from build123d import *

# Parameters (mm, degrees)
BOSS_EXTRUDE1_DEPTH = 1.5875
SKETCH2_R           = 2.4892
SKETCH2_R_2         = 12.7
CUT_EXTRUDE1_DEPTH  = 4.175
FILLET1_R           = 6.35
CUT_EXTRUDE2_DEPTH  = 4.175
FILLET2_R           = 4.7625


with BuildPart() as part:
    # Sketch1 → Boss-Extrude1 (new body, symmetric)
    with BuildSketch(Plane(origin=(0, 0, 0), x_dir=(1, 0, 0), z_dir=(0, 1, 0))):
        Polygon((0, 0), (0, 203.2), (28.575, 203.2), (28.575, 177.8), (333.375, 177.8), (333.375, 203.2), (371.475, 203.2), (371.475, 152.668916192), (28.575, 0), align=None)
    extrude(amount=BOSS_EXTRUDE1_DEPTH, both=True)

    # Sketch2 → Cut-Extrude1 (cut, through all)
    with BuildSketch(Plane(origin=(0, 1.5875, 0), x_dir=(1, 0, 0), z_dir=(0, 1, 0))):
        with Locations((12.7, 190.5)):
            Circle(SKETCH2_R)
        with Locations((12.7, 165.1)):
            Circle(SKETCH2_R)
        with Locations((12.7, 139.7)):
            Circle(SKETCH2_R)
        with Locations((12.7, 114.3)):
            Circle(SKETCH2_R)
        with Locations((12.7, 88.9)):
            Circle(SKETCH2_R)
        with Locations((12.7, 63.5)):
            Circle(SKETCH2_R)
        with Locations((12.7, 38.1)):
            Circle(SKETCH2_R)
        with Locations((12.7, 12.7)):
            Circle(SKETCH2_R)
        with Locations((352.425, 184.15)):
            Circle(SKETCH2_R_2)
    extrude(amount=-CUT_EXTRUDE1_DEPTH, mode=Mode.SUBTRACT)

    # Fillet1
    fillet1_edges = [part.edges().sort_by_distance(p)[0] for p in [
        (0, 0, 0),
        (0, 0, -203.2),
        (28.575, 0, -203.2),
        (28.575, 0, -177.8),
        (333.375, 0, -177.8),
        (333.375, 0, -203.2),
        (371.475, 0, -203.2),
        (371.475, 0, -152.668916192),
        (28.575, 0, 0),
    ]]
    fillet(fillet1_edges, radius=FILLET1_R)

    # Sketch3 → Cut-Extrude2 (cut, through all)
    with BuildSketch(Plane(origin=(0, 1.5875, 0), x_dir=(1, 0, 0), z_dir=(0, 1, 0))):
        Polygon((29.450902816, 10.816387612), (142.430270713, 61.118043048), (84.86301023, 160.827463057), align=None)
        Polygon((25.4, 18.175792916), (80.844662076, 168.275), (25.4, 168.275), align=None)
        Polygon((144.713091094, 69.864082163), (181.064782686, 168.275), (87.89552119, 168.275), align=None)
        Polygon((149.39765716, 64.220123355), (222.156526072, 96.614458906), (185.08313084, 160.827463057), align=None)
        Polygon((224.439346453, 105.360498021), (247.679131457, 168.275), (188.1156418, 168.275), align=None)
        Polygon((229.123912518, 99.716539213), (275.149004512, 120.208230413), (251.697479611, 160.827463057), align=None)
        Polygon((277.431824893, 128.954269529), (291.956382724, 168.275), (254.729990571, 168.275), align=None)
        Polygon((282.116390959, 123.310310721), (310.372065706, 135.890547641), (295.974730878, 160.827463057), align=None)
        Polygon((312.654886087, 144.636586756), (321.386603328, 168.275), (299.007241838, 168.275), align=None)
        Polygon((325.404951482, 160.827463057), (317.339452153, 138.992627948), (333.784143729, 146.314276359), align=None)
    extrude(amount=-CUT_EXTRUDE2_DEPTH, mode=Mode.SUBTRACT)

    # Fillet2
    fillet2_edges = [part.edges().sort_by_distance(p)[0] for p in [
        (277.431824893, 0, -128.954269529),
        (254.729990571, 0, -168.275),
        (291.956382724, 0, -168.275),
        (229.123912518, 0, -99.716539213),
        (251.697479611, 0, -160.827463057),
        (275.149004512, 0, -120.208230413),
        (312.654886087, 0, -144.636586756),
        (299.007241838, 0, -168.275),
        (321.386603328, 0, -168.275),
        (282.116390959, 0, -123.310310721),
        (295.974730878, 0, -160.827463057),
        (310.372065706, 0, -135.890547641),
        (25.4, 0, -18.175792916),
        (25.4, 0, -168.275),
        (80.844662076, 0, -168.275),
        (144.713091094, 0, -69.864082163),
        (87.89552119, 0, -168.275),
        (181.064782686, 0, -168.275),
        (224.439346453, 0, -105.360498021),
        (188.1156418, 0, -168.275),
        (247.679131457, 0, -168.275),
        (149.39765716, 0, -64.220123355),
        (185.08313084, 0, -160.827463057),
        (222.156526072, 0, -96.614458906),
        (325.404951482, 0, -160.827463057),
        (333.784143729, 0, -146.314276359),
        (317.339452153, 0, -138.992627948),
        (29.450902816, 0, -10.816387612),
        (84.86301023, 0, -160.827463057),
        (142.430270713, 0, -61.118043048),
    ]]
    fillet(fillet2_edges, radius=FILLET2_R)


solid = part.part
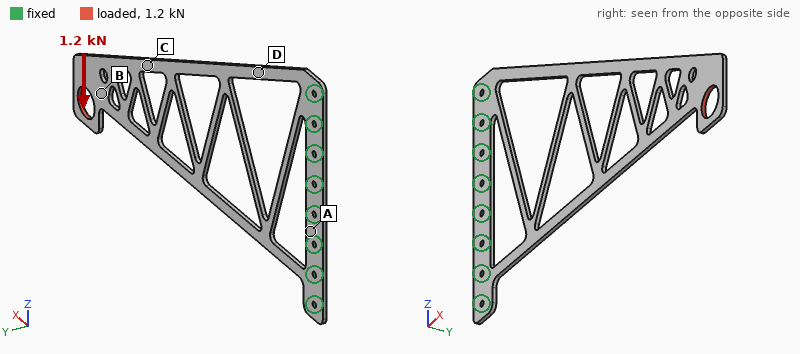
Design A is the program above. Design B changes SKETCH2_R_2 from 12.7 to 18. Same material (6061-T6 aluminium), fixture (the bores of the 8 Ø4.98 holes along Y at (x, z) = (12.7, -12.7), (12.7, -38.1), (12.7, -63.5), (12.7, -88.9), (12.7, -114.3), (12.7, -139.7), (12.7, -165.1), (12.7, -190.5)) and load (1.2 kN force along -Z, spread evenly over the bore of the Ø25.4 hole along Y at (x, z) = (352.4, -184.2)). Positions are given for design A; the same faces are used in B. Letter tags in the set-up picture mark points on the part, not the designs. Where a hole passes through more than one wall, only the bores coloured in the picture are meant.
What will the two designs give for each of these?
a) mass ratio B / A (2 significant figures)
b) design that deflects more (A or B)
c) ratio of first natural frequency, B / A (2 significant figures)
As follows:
0.97
B
1.1
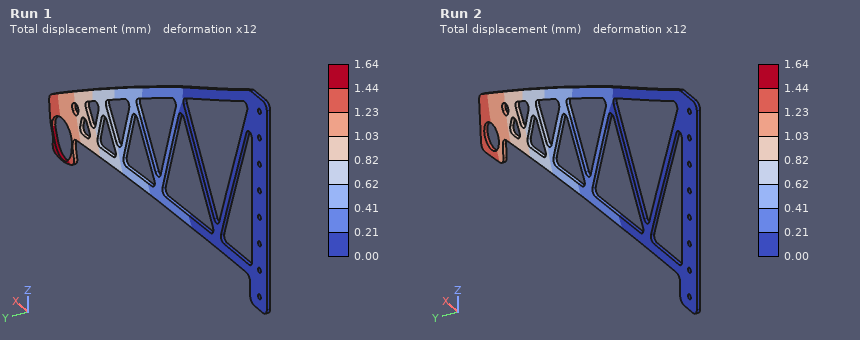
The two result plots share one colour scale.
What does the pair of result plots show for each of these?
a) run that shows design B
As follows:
Run 1
